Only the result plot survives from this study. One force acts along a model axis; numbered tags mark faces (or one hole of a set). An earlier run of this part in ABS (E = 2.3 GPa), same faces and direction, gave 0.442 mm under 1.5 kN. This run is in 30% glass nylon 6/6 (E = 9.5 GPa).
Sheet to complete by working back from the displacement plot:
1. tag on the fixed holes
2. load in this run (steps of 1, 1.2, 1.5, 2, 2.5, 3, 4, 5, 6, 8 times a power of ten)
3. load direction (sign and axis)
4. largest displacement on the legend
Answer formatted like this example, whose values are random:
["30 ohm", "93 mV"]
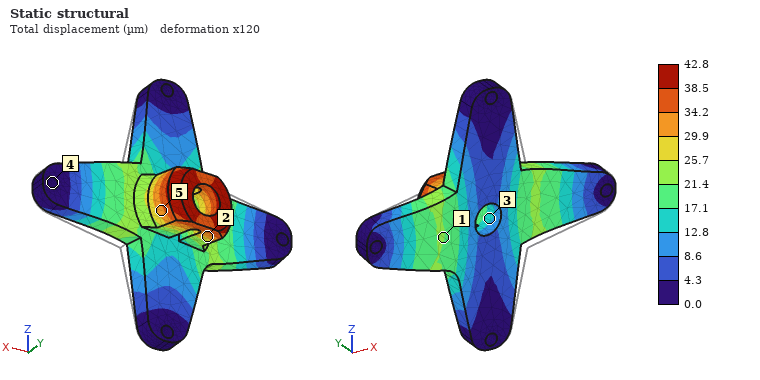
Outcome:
["4", "600 N", "-X", "42.8 µm"]
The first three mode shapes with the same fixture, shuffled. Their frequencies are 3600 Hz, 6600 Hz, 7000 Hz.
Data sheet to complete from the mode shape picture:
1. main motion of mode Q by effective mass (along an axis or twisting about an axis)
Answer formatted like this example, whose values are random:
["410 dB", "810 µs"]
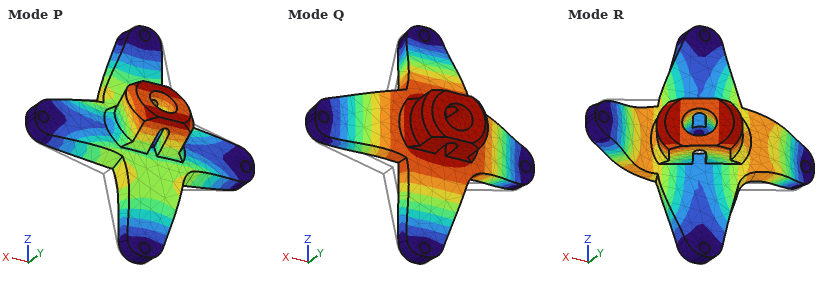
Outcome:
["along Y"]
